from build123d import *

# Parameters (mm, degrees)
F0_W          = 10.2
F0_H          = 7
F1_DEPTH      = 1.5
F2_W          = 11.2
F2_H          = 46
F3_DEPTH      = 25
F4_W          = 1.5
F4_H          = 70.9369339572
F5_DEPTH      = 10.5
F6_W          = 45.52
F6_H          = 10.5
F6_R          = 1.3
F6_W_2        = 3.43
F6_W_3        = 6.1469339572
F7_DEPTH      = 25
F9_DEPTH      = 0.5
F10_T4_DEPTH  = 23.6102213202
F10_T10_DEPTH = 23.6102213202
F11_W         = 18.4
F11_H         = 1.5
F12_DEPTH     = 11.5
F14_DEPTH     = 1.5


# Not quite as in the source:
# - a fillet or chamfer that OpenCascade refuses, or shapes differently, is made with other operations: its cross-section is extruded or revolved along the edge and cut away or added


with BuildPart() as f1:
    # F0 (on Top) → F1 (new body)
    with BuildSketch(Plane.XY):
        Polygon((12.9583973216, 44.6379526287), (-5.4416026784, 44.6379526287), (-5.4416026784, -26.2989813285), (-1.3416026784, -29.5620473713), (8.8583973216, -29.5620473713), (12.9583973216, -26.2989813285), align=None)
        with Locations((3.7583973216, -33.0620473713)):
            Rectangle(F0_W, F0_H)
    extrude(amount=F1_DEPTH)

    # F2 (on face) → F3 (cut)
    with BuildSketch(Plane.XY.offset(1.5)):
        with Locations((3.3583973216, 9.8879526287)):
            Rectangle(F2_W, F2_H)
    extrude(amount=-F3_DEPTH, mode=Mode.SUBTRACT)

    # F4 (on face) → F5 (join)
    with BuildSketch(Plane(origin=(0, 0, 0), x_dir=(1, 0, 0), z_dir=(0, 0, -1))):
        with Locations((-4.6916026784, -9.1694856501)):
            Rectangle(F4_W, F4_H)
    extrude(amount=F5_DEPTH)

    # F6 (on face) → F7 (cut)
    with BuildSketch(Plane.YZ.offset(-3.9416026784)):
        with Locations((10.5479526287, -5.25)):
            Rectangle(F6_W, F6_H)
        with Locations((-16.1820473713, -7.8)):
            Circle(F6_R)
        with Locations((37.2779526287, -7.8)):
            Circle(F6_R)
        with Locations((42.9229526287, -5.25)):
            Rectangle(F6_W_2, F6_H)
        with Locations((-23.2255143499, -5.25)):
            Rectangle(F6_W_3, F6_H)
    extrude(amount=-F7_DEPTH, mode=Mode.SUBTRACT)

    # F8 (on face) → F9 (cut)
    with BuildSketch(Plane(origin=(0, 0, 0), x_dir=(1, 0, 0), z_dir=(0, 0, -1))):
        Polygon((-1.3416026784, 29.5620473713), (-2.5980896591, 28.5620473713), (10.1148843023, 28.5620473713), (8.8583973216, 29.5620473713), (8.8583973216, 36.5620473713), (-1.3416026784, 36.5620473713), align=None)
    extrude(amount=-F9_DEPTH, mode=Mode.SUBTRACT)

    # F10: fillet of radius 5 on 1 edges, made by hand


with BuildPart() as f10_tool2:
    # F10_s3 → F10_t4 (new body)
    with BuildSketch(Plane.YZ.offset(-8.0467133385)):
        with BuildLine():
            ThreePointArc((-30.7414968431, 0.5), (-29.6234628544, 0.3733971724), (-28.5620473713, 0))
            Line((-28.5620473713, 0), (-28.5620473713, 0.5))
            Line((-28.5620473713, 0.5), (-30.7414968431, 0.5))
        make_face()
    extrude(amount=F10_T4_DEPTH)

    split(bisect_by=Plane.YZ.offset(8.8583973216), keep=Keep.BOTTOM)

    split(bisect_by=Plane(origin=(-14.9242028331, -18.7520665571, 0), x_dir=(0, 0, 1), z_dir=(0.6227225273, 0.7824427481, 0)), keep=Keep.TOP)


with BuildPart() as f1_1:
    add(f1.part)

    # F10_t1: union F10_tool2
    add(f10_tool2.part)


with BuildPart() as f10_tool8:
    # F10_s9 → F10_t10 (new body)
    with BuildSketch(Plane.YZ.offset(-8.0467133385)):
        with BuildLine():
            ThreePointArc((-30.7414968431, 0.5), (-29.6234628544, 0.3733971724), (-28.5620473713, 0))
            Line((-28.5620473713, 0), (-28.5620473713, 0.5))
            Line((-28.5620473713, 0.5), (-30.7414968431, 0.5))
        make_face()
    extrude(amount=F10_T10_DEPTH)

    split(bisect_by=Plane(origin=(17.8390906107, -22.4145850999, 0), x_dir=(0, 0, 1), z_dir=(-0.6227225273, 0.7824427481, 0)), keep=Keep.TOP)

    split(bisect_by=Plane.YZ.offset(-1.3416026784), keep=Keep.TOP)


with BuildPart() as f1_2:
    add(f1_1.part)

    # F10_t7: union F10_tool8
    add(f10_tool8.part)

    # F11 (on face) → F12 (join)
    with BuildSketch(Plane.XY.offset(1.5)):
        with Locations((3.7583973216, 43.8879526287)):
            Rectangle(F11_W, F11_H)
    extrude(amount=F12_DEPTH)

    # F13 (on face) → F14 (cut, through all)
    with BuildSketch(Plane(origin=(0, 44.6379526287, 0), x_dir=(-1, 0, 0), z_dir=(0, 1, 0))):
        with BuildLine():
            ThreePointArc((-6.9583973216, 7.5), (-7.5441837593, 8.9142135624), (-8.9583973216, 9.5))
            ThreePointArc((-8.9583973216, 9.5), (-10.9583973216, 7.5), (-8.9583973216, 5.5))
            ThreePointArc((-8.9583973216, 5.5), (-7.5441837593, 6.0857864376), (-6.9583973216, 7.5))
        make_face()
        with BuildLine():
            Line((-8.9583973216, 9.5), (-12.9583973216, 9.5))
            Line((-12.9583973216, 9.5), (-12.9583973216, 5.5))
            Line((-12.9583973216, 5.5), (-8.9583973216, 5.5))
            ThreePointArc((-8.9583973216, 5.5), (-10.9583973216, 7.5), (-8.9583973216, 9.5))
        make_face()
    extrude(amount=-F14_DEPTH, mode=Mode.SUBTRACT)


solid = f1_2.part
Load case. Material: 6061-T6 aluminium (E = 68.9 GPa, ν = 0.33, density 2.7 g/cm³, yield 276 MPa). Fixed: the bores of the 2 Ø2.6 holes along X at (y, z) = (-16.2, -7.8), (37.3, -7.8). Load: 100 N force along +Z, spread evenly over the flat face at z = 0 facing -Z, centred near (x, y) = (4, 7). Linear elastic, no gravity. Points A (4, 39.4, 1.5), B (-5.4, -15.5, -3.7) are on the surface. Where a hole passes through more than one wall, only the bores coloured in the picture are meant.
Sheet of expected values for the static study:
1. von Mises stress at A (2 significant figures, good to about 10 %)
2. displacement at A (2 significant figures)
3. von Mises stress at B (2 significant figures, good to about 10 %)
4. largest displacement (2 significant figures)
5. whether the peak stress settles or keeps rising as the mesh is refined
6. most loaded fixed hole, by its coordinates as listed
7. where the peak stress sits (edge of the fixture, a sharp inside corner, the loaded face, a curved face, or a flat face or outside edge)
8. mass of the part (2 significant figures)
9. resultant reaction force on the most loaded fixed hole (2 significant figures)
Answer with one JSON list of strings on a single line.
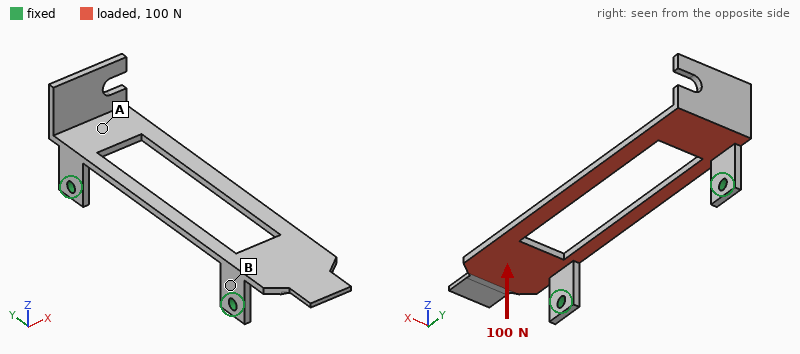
["28 MPa", "0.23 mm", "140 MPa", "0.69 mm", "keeps rising", "(-16.2, -7.8)", "edge of the fixture", "5.0 g", "55 N"]
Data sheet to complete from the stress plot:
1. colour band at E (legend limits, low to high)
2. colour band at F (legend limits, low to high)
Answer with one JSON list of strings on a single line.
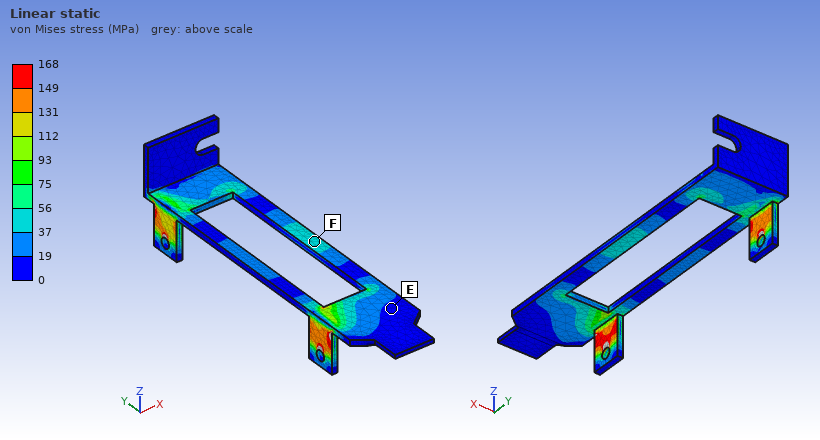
["0 to 19 MPa", "37 to 56 MPa"]
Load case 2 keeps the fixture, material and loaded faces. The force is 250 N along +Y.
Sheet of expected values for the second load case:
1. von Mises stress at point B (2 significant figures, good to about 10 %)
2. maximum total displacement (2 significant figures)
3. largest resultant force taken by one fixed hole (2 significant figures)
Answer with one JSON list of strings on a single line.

["58 MPa", "0.27 mm", "130 N"]
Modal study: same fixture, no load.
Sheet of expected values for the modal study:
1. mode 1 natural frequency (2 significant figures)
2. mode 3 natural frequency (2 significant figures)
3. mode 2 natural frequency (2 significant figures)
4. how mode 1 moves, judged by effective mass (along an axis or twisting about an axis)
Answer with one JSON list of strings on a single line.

["1100 Hz", "2300 Hz", "1500 Hz", "along Z"]
